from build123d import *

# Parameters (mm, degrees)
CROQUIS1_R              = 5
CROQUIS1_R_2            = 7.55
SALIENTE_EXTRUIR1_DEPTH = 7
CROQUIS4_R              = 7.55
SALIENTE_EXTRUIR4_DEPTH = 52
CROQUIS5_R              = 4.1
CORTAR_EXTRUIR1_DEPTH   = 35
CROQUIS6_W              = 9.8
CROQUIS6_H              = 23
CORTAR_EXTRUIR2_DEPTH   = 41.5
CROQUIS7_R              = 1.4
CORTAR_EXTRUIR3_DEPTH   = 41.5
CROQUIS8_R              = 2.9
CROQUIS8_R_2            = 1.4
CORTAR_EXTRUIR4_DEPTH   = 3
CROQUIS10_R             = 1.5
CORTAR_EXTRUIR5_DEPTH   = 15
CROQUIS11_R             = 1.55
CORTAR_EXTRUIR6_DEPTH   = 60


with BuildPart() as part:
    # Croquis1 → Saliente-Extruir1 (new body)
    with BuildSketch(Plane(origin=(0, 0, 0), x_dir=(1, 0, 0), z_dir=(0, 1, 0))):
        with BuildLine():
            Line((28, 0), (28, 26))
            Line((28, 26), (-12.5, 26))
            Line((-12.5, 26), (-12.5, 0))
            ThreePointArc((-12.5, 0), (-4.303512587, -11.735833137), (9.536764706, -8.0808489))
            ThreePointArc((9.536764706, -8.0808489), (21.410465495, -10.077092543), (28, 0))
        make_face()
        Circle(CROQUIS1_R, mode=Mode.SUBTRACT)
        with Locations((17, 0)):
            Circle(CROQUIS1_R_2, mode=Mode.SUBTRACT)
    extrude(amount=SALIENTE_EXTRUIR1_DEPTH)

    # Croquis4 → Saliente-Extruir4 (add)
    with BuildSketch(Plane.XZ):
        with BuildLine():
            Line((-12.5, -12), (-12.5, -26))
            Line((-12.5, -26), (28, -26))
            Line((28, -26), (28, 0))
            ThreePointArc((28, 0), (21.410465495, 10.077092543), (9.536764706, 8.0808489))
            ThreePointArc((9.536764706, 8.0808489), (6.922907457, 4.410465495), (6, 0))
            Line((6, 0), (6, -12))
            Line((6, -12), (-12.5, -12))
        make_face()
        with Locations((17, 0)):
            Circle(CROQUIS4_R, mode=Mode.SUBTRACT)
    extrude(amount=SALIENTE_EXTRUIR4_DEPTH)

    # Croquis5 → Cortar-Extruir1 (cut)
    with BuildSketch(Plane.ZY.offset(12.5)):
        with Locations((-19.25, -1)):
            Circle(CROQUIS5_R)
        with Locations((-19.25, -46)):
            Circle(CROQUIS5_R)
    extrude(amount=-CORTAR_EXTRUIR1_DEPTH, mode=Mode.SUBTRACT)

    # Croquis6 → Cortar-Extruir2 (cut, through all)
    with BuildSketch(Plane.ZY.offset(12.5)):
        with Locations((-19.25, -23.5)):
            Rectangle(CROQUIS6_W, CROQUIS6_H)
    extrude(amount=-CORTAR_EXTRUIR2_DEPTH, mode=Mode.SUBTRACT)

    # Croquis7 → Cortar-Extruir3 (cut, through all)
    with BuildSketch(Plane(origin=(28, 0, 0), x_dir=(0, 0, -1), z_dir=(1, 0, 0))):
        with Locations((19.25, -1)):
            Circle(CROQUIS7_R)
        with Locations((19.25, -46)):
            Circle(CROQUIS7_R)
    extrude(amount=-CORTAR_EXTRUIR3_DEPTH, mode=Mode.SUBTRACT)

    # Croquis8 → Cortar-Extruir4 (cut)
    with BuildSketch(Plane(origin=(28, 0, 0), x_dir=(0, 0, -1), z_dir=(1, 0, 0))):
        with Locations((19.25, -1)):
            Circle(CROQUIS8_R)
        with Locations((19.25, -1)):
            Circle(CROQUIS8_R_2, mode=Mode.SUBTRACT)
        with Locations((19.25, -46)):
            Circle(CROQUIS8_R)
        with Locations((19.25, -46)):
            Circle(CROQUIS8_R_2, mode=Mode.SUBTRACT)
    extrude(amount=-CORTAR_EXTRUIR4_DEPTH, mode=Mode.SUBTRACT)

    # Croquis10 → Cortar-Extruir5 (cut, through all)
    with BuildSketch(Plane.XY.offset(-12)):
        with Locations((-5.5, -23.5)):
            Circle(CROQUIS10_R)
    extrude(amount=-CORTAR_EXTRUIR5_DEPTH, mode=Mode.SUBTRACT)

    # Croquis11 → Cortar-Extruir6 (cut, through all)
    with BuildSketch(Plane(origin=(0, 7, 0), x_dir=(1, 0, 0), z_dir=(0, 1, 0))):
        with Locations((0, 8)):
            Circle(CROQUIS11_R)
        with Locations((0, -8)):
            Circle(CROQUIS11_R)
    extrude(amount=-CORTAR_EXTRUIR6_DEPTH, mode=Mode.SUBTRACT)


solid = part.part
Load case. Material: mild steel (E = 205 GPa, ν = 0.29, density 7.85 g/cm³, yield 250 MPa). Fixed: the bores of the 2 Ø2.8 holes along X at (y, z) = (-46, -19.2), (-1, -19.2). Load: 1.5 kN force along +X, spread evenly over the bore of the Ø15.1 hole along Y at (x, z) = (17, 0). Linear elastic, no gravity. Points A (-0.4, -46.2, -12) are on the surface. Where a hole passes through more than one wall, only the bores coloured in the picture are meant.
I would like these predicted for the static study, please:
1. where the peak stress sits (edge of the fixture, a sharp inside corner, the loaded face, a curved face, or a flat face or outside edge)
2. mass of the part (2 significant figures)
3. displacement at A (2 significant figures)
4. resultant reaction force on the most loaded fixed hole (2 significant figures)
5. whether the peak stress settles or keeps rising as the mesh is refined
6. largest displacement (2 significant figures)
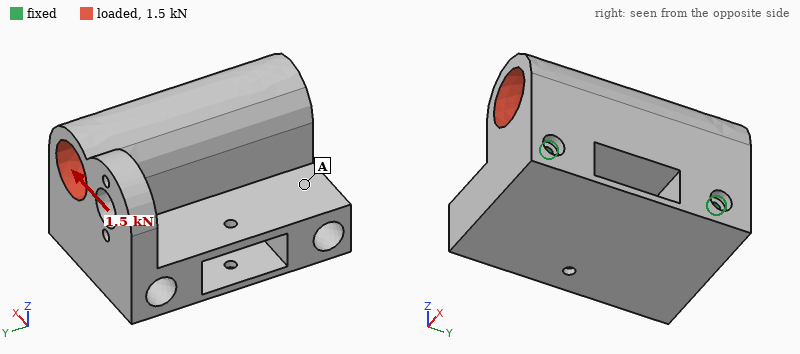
edge of the fixture
310 g
0.11 mm
790 N
keeps rising
0.18 mm
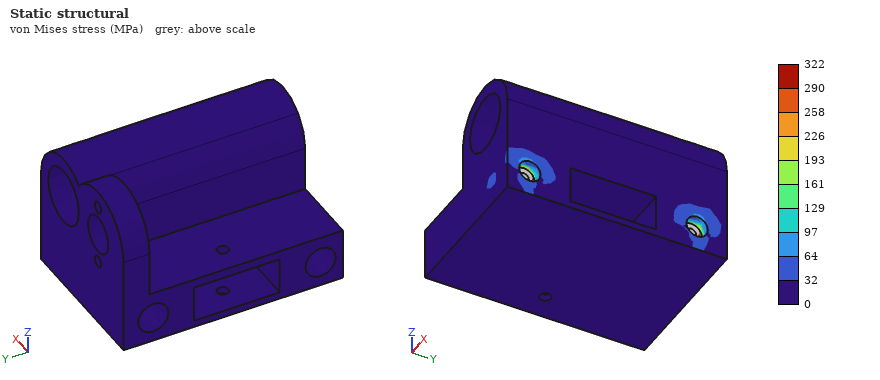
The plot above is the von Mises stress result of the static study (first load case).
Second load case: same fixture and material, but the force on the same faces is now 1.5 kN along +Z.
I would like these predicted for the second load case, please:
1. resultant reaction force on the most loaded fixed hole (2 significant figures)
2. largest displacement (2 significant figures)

790 N
64 µm
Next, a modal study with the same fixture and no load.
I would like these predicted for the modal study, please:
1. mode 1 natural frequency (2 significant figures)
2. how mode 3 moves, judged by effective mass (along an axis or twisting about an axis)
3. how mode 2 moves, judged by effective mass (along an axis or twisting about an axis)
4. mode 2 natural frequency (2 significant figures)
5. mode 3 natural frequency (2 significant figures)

1100 Hz
along Y
along Y
7100 Hz
8000 Hz
